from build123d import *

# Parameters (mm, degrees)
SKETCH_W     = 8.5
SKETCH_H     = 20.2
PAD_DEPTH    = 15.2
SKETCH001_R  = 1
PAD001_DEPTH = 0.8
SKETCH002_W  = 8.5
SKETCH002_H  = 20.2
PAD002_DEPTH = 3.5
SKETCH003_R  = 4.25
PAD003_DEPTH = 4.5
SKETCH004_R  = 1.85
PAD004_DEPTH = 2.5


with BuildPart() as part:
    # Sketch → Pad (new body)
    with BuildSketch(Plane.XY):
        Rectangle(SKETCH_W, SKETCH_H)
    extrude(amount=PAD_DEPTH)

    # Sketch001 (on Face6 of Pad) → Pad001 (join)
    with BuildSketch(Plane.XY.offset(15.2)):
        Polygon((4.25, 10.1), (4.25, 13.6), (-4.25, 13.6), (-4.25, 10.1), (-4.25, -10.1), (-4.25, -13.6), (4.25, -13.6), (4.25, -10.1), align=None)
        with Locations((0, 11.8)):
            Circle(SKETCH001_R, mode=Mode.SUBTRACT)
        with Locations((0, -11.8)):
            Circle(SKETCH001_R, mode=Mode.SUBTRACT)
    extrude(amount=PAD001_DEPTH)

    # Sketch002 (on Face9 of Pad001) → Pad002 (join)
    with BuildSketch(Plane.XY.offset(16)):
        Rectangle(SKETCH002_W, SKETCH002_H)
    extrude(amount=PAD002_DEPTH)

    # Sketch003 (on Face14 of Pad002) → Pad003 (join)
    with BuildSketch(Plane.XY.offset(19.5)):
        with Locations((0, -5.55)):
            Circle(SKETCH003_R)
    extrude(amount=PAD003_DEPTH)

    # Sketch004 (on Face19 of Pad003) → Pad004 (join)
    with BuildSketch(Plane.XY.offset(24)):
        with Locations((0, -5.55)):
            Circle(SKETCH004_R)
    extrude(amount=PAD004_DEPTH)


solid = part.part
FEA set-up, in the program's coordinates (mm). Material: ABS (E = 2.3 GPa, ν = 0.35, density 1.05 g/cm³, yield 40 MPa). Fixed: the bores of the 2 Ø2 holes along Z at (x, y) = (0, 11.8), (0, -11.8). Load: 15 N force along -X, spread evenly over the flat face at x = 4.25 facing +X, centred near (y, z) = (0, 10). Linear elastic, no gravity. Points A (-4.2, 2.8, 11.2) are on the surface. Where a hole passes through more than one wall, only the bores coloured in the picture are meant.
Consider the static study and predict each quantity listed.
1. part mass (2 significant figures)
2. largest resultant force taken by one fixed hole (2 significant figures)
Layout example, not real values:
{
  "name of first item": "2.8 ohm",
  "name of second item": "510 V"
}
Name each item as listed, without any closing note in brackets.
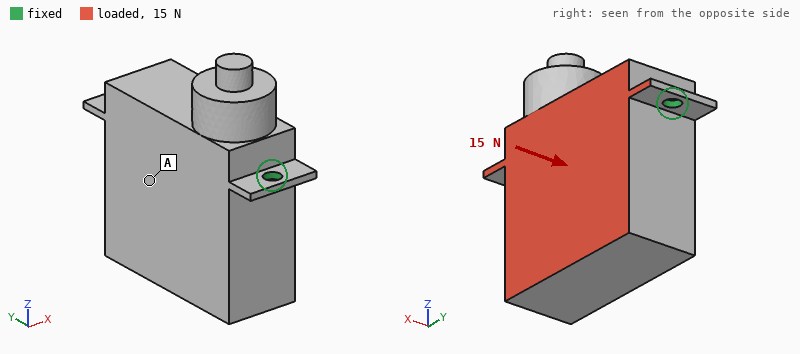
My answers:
{
  "part mass": "3.9 g",
  "largest resultant force taken by one fixed hole": "7.5 N"
}
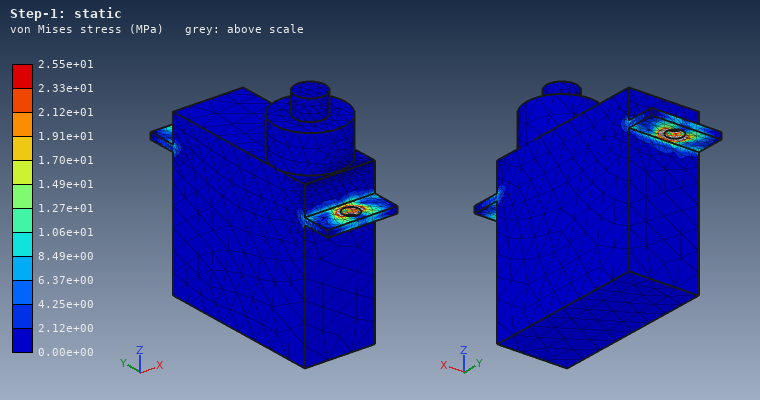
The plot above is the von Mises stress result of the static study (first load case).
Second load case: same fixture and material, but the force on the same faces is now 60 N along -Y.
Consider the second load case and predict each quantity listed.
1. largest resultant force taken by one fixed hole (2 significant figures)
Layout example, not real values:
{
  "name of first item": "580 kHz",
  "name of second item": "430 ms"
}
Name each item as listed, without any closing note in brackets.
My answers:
{
  "largest resultant force taken by one fixed hole": "36 N"
}
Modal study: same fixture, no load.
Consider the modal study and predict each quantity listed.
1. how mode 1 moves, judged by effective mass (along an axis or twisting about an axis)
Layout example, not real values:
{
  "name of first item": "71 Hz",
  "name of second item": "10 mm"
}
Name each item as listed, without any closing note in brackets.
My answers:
{
  "how mode 1 moves, judged by effective mass": "along X"
}
